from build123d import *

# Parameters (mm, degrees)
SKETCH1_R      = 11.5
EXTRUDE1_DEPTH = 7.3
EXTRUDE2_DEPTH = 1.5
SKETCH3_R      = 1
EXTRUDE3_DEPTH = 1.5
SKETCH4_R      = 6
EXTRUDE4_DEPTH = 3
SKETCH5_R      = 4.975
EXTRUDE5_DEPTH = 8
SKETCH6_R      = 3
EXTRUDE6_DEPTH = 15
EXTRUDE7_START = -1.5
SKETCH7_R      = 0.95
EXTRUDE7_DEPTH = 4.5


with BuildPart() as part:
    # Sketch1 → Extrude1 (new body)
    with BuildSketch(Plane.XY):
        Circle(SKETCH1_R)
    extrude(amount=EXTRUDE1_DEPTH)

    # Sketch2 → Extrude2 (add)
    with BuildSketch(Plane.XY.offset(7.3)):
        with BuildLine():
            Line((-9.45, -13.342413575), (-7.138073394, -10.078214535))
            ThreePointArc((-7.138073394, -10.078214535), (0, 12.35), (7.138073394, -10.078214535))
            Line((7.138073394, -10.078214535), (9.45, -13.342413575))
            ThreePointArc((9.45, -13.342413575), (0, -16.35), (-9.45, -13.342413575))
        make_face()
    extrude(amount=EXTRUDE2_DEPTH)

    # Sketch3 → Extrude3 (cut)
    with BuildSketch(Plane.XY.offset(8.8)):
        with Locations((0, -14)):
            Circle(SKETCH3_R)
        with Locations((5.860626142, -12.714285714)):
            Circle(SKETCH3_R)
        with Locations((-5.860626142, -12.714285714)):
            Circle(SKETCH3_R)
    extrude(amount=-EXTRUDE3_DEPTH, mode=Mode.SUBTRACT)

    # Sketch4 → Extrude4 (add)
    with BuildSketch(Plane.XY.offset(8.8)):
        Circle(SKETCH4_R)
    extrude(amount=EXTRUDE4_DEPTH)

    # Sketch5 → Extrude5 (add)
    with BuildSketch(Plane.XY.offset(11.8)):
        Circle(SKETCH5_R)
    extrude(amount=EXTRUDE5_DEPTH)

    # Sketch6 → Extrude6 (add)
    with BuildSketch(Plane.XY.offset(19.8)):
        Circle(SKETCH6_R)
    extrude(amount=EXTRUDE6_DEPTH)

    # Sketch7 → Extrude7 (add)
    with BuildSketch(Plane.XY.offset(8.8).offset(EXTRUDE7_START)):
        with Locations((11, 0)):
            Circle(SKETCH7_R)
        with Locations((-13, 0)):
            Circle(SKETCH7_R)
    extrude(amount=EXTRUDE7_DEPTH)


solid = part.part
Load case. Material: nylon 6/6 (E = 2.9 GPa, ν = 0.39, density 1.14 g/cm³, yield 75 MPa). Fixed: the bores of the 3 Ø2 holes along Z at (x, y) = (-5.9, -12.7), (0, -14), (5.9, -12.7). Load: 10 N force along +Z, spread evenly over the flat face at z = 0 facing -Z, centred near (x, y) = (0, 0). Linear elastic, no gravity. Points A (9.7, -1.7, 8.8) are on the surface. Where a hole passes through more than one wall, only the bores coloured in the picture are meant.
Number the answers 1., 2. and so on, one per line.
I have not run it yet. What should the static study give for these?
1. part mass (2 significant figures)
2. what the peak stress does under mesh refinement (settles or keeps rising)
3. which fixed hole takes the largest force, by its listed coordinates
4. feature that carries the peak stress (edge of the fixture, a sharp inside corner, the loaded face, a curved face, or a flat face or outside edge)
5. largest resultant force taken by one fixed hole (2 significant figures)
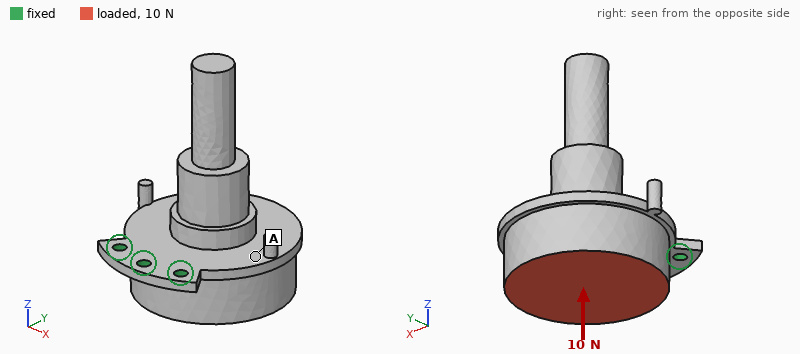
1. 6.0 g
2. keeps rising
3. (0, -14)
4. edge of the fixture
5. 15 N
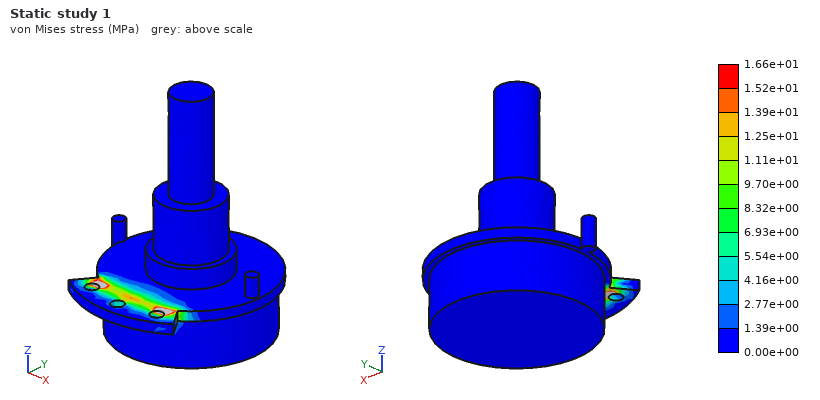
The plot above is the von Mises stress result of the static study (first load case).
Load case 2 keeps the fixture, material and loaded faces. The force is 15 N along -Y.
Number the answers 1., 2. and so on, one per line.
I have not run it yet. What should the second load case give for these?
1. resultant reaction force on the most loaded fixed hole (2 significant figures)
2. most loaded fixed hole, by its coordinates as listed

1. 22 N
2. (0, -14)
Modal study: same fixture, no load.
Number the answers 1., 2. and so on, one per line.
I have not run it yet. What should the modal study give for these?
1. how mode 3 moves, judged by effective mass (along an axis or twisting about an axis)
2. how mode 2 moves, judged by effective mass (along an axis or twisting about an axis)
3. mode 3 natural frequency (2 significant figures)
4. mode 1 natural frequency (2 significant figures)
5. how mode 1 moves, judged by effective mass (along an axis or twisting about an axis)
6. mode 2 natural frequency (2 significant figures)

1. along X
2. along X
3. 2500 Hz
4. 360 Hz
5. along Z
6. 1600 Hz
